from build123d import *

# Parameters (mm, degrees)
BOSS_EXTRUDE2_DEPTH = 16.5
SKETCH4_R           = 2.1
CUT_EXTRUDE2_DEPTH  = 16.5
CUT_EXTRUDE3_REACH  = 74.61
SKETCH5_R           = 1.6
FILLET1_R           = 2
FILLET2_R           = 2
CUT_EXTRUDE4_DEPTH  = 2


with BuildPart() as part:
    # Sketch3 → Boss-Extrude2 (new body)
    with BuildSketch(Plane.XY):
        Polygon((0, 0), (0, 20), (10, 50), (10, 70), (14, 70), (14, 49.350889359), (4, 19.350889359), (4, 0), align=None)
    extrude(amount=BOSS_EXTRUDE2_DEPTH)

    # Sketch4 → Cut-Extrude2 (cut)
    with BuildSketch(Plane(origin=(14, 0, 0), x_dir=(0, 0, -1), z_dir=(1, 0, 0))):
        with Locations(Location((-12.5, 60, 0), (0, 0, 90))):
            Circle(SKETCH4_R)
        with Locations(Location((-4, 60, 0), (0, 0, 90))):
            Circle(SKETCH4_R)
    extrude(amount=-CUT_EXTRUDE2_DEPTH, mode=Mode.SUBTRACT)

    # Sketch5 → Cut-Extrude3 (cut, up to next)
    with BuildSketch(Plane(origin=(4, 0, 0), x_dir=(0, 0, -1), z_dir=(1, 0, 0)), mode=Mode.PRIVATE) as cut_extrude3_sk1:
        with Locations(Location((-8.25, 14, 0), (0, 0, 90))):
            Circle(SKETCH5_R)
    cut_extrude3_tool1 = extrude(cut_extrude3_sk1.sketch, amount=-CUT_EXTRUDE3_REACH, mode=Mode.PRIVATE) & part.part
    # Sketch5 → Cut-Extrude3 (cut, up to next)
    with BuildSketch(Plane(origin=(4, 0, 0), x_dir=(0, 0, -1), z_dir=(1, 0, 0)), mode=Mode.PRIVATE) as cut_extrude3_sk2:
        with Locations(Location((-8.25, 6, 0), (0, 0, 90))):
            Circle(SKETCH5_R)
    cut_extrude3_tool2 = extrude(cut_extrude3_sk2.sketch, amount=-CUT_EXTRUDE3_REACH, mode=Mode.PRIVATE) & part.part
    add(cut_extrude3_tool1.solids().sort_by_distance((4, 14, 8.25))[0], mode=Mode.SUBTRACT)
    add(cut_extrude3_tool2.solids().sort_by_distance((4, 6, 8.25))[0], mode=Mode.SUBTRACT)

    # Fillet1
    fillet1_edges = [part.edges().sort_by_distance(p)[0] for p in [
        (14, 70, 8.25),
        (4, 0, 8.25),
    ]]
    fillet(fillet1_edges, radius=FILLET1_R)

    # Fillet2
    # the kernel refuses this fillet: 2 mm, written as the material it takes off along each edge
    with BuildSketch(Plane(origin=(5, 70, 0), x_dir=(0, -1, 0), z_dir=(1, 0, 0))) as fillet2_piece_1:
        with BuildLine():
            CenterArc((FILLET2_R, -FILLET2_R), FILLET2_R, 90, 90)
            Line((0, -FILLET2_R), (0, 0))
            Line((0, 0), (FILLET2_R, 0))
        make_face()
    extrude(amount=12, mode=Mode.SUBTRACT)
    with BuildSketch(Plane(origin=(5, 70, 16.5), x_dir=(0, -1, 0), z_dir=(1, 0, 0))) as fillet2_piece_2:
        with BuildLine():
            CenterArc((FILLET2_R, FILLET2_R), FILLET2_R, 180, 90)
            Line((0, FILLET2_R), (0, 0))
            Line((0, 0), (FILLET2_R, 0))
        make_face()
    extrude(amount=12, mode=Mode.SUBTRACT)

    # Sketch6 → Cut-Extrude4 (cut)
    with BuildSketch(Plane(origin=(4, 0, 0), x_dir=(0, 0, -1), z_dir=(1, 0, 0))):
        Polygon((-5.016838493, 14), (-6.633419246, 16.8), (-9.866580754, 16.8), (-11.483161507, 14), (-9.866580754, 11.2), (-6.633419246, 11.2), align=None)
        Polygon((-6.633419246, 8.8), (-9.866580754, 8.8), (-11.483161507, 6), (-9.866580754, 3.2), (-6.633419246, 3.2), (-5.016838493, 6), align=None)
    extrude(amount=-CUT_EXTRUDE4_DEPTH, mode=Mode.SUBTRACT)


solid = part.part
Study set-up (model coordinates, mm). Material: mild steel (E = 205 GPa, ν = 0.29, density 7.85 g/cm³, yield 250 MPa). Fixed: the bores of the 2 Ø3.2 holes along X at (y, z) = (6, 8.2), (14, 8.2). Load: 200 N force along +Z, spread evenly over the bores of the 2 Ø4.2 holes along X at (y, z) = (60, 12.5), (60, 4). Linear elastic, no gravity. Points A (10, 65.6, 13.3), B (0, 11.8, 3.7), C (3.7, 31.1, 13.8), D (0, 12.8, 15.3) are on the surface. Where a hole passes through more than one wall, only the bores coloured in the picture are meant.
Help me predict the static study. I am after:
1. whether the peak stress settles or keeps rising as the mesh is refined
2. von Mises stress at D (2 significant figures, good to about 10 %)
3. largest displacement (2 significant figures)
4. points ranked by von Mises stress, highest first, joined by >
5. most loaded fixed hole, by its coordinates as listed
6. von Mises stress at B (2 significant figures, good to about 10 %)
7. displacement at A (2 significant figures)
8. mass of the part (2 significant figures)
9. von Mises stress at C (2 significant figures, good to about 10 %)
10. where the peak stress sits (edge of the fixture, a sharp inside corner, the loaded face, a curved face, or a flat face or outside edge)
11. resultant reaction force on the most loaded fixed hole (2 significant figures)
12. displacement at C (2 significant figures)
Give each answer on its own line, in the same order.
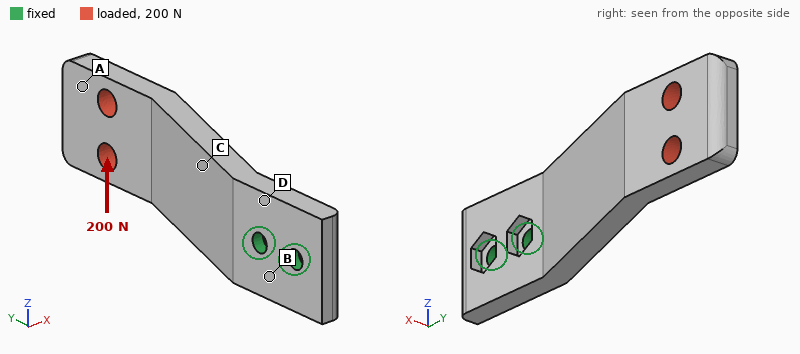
keeps rising
51 MPa
66 µm
B > D > C > A
(14, 8.2)
71 MPa
59 µm
35 g
26 MPa
edge of the fixture
950 N
15 µm
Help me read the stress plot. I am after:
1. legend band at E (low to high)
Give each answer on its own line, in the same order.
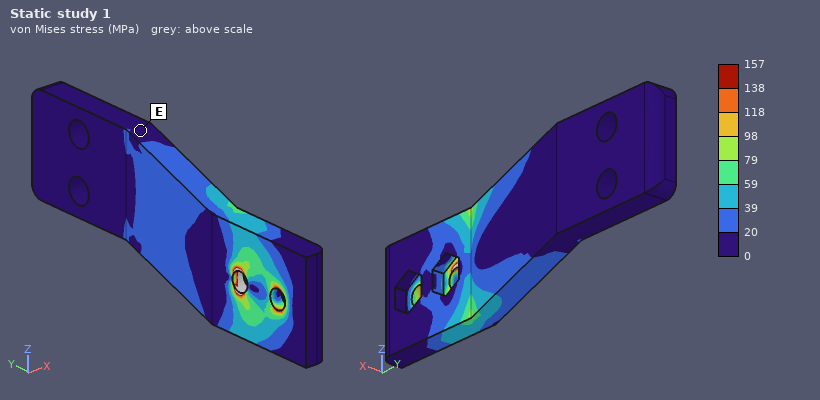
0 to 20 MPa
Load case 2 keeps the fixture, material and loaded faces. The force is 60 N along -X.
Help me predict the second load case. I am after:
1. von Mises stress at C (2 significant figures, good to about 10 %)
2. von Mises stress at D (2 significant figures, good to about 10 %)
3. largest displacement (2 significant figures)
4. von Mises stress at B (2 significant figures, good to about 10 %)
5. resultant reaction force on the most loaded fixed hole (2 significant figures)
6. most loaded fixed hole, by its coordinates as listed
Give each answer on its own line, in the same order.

40 MPa
38 MPa
0.18 mm
23 MPa
350 N
(14, 8.2)
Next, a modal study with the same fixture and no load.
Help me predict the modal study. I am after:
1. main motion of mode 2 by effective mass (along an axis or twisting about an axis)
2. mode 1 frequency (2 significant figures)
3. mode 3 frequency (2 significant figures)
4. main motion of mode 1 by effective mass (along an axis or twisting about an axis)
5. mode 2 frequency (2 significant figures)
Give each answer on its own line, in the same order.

along Z
950 Hz
5400 Hz
along X
2700 Hz
